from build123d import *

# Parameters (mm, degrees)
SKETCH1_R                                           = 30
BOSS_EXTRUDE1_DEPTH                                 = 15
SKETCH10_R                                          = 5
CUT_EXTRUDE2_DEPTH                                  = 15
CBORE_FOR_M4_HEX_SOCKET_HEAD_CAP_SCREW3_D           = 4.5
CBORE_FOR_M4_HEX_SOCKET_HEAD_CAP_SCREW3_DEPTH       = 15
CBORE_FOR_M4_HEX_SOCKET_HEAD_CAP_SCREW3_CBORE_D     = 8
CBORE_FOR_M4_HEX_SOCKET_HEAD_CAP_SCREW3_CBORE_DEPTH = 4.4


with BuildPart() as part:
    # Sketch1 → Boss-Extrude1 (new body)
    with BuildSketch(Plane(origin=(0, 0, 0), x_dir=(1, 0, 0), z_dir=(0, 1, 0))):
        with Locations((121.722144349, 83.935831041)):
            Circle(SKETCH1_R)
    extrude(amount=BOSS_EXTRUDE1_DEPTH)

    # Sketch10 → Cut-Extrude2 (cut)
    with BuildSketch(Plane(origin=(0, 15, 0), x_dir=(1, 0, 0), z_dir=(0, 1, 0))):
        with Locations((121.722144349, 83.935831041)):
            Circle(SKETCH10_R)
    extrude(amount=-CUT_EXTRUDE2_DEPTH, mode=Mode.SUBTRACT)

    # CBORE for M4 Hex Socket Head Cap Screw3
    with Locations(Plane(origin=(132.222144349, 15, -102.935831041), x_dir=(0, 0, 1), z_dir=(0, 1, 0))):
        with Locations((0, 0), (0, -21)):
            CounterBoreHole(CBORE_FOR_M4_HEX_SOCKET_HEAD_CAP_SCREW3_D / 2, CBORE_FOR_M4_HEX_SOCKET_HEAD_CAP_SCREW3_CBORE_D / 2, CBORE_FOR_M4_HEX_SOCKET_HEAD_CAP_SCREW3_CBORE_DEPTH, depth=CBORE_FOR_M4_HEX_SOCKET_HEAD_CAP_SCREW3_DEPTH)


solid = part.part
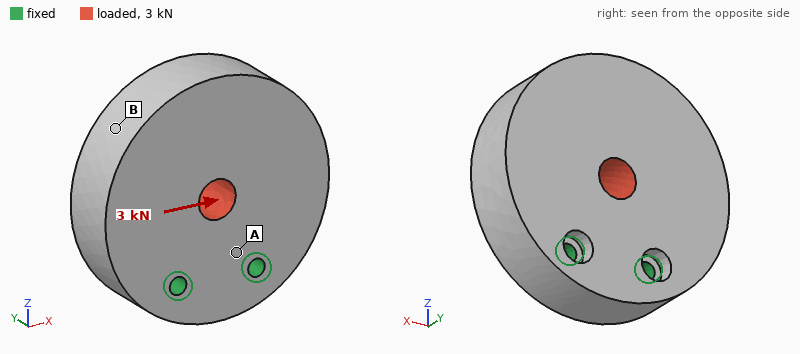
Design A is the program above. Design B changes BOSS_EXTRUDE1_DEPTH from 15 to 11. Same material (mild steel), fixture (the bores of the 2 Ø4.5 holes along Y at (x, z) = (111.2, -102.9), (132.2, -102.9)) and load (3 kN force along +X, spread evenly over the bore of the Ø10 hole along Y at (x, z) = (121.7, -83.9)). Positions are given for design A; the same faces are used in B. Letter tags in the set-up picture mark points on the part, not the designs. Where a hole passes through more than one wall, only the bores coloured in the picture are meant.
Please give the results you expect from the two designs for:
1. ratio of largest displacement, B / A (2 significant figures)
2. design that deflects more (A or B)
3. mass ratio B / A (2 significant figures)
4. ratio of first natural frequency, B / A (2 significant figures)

1.2
B
0.74
0.96
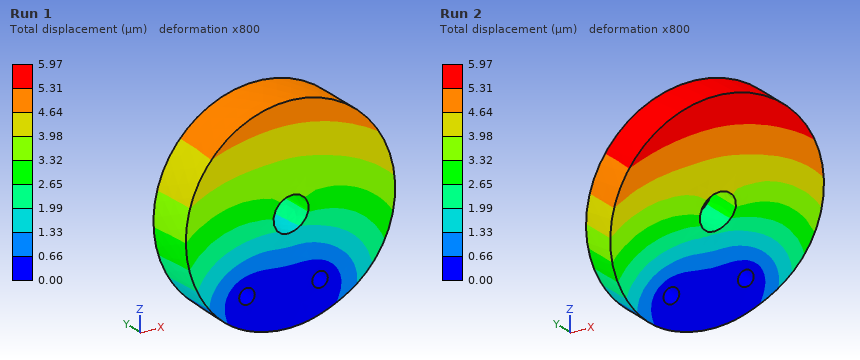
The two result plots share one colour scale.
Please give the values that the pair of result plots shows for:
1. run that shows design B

Run 2
